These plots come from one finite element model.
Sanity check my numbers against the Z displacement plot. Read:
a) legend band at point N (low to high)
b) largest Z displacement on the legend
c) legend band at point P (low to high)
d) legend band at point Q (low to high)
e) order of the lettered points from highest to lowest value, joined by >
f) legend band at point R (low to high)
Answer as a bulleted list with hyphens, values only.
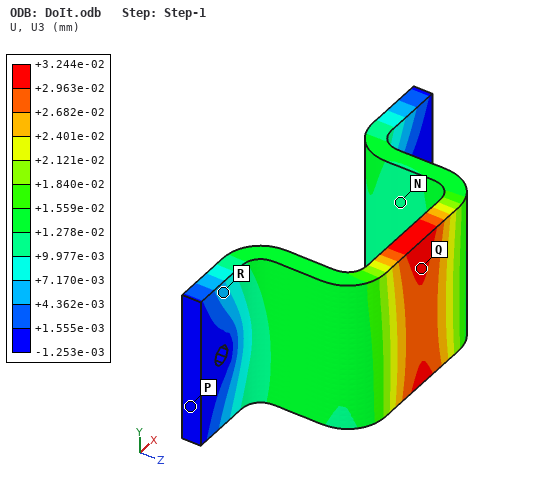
- +9.977e-03 to +1.278e-02 mm
- +3.244e-02 mm
- -1.253e-03 to +1.555e-03 mm
- +2.963e-02 to +3.244e-02 mm
- Q > N > R > P
- +4.362e-03 to +7.170e-03 mm
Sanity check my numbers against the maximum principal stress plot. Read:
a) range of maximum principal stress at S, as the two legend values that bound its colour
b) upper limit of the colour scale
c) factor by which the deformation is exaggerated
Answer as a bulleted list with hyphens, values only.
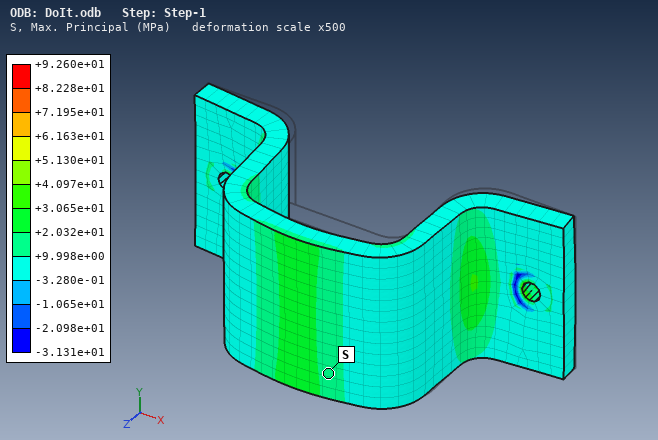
- +9.998e+00 to +2.032e+01 MPa
- +9.260e+01 MPa
- 500
